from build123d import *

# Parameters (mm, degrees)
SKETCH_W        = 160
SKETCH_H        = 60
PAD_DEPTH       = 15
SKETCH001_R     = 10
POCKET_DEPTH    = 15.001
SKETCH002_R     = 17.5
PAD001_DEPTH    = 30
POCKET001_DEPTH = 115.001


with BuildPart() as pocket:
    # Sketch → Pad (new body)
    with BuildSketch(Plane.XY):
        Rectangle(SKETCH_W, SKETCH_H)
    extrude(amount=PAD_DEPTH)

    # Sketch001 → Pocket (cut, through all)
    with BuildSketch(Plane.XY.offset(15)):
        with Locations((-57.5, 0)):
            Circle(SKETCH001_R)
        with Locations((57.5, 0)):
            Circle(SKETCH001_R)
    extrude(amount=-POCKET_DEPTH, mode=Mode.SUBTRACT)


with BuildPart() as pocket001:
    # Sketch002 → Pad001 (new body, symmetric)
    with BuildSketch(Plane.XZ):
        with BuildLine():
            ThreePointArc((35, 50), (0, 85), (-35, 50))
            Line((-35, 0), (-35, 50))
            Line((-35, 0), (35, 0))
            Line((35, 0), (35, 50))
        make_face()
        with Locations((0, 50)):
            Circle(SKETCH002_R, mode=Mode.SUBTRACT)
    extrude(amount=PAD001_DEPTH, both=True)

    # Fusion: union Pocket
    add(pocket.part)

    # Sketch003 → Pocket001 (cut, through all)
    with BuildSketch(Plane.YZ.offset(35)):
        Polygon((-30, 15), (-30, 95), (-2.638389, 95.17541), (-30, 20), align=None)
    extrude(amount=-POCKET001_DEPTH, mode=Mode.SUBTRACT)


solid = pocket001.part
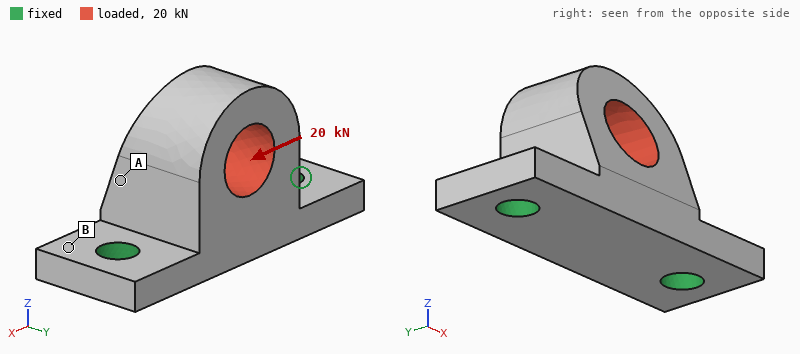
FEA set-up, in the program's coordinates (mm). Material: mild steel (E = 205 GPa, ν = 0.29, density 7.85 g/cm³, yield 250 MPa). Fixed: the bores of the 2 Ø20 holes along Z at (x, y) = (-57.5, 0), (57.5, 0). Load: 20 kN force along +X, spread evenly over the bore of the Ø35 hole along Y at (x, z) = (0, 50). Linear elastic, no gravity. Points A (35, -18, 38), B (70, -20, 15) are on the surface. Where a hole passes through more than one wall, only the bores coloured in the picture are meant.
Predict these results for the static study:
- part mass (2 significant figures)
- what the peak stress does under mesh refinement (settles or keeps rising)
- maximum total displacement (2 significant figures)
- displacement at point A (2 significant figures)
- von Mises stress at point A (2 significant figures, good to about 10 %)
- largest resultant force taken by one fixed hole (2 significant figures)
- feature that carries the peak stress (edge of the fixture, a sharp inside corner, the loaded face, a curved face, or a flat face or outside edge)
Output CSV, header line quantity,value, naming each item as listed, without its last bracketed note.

quantity,value
part mass,2.4 kg
what the peak stress does under mesh refinement,keeps rising
maximum total displacement,25 µm
displacement at point A,12 µm
von Mises stress at point A,17 MPa
largest resultant force taken by one fixed hole,14 kN
feature that carries the peak stress,edge of the fixture
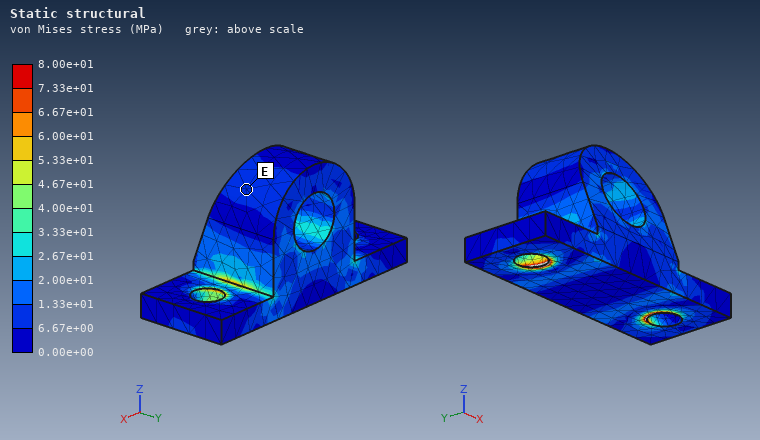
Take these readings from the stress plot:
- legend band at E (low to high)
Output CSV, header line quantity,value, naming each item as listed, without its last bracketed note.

quantity,value
legend band at E,6.67e+00 to 1.33e+01 MPa
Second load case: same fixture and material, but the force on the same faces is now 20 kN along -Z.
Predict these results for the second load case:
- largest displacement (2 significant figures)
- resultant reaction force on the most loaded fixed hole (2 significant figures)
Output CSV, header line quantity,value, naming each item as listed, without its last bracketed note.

quantity,value
largest displacement,22 µm
resultant reaction force on the most loaded fixed hole,11 kN
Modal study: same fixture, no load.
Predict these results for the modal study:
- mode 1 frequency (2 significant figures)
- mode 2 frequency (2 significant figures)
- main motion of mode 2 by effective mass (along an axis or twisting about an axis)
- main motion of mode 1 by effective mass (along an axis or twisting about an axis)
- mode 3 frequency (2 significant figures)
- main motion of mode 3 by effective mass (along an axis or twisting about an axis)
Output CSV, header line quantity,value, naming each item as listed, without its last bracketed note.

quantity,value
mode 1 frequency,2200 Hz
mode 2 frequency,4800 Hz
main motion of mode 2 by effective mass,along X
main motion of mode 1 by effective mass,along Y
mode 3 frequency,5300 Hz
main motion of mode 3 by effective mass,along Z
